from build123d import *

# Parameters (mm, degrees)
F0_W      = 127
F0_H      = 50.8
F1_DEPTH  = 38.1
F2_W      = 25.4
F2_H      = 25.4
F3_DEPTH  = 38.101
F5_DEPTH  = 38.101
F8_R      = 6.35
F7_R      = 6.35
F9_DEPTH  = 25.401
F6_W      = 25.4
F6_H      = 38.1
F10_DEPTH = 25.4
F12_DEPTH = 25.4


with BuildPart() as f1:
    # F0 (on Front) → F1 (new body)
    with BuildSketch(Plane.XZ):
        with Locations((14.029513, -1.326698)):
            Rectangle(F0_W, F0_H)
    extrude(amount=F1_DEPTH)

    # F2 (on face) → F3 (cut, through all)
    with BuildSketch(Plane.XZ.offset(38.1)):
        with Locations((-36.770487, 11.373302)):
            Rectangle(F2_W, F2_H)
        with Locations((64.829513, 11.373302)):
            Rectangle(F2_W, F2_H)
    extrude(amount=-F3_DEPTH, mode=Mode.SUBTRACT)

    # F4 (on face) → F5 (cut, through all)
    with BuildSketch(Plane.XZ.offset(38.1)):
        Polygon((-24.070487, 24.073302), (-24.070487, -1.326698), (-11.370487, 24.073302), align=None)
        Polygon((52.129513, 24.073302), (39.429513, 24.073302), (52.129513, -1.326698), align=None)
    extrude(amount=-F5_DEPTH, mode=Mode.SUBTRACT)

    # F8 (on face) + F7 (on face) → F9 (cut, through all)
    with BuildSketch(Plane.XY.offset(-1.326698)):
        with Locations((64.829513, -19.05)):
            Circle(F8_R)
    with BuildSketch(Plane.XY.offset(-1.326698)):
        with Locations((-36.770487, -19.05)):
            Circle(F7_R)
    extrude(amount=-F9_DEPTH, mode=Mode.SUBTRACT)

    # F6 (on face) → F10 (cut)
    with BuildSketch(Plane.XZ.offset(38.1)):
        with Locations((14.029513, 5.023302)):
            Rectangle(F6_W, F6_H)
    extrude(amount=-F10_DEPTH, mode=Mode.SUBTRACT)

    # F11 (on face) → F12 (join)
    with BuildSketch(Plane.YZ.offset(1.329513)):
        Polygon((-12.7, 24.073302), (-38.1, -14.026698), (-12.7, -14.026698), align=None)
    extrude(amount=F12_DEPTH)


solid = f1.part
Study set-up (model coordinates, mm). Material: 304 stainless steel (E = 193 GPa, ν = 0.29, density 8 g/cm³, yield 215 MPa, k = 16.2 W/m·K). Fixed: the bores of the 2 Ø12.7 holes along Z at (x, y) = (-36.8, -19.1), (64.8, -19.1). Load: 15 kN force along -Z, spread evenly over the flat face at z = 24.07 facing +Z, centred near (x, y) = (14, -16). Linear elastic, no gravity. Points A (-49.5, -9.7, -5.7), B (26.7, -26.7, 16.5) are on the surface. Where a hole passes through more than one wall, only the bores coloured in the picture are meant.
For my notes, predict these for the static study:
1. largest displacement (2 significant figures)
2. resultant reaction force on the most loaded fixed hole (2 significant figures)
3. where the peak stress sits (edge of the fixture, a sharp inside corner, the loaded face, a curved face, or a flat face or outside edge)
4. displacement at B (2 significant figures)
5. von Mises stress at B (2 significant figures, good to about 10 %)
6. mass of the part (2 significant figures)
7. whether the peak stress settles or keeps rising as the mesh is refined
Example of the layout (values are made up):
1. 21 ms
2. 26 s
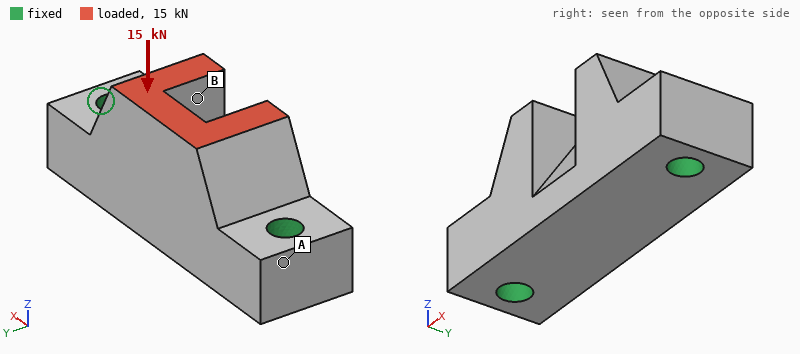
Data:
1. 9.0 µm
2. 8.0 kN
3. edge of the fixture
4. 6.4 µm
5. 14 MPa
6. 1.3 kg
7. keeps rising
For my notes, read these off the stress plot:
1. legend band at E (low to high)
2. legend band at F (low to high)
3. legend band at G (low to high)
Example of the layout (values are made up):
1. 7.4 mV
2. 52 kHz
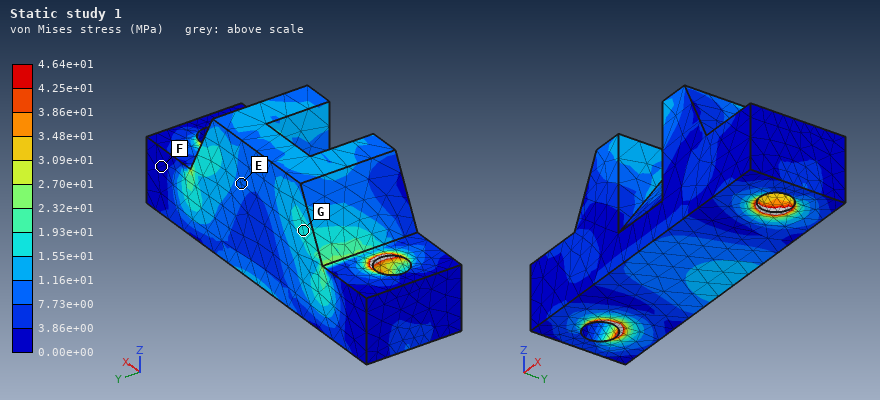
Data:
1. 7.73e+00 to 1.16e+01 MPa
2. 0.00e+00 to 3.86e+00 MPa
3. 1.55e+01 to 1.93e+01 MPa
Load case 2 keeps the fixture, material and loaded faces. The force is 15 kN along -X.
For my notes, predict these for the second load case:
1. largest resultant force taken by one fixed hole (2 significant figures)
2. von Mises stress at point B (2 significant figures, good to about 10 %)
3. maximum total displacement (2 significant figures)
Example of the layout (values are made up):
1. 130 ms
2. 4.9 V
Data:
1. 9.8 kN
2. 24 MPa
3. 11 µm
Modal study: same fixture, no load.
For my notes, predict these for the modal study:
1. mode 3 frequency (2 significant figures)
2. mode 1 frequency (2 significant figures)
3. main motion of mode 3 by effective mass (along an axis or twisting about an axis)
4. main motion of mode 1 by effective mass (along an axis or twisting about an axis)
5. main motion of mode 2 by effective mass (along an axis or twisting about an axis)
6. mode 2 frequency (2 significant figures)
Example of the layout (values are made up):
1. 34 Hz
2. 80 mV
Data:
1. 11 kHz
2. 6400 Hz
3. along Y
4. along Y
5. along Z
6. 9400 Hz
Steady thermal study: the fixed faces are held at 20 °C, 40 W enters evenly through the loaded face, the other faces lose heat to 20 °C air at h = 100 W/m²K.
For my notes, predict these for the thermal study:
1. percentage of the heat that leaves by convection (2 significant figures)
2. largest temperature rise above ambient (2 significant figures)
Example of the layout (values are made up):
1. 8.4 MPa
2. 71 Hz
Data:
1. 61 %
2. 47 K
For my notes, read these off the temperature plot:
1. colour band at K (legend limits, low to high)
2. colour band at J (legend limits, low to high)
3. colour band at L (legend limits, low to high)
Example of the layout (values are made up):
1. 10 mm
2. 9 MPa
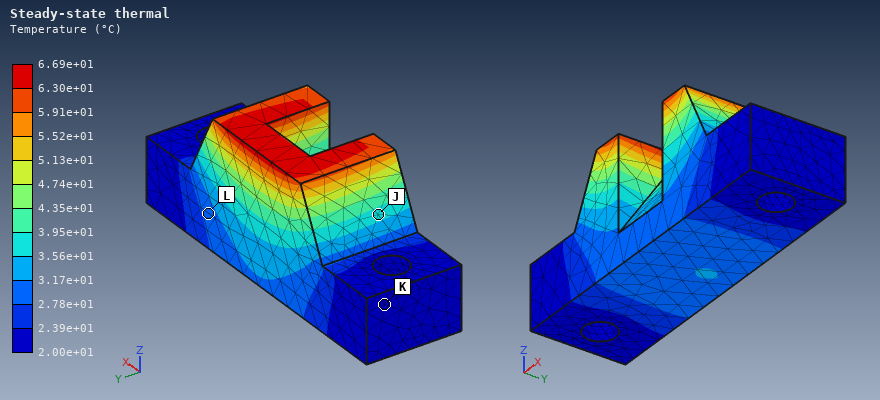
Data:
1. 2.00e+01 to 2.39e+01 °C
2. 3.56e+01 to 3.95e+01 °C
3. 2.78e+01 to 3.17e+01 °C
